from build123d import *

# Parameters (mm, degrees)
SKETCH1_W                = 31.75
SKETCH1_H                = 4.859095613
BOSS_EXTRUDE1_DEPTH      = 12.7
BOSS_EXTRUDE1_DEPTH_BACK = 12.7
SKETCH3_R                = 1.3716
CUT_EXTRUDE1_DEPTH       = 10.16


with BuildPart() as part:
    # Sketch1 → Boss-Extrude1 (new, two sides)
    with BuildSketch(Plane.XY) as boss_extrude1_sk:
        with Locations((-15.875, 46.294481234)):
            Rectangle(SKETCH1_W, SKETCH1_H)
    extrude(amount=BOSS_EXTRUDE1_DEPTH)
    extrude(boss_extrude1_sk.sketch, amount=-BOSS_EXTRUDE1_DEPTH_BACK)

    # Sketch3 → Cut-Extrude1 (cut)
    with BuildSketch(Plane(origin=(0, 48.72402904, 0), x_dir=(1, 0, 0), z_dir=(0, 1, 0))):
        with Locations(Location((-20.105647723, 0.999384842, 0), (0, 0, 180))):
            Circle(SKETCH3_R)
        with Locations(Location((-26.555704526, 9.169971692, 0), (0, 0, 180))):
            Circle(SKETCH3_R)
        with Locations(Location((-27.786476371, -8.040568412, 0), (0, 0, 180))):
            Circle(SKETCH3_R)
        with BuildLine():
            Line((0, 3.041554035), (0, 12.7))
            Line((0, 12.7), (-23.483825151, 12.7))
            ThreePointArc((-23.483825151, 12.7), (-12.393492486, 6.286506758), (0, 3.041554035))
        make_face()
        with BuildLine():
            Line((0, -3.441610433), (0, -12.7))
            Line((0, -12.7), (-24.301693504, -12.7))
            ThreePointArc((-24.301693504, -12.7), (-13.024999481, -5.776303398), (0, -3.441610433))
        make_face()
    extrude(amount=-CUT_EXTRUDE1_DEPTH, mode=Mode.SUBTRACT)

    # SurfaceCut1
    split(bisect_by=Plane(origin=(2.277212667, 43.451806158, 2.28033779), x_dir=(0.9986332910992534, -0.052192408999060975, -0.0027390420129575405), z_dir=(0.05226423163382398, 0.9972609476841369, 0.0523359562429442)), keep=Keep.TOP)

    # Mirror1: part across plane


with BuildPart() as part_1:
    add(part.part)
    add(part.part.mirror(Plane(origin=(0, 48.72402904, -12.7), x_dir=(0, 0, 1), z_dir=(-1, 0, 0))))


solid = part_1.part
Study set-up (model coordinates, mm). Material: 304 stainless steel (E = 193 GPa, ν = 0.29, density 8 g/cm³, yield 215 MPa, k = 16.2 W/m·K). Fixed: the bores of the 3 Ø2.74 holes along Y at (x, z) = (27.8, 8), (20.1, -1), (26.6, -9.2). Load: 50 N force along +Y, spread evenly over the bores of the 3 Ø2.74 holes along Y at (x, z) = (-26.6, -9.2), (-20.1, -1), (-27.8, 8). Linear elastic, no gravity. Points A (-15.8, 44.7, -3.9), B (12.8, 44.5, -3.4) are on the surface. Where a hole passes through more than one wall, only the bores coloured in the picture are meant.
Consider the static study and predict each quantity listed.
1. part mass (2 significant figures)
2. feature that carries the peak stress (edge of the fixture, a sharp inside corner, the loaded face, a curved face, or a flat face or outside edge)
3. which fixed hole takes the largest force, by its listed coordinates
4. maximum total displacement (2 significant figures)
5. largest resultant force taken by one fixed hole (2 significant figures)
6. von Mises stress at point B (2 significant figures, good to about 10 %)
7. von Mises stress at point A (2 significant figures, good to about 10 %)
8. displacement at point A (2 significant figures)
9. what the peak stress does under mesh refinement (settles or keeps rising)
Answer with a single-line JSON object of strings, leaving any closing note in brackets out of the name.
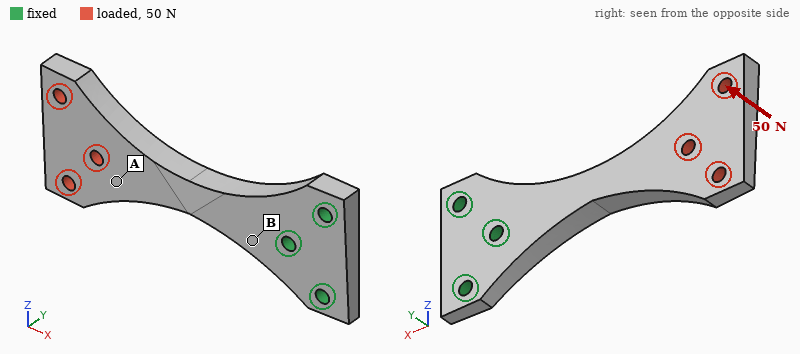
{"part mass": "31 g", "feature that carries the peak stress": "edge of the fixture", "which fixed hole takes the largest force, by its listed coordinates": "(20.1, -1)", "maximum total displacement": "0.13 mm", "largest resultant force taken by one fixed hole": "160 N", "von Mises stress at point B": "48 MPa", "von Mises stress at point A": "10 MPa", "displacement at point A": "0.073 mm", "what the peak stress does under mesh refinement": "keeps rising"}
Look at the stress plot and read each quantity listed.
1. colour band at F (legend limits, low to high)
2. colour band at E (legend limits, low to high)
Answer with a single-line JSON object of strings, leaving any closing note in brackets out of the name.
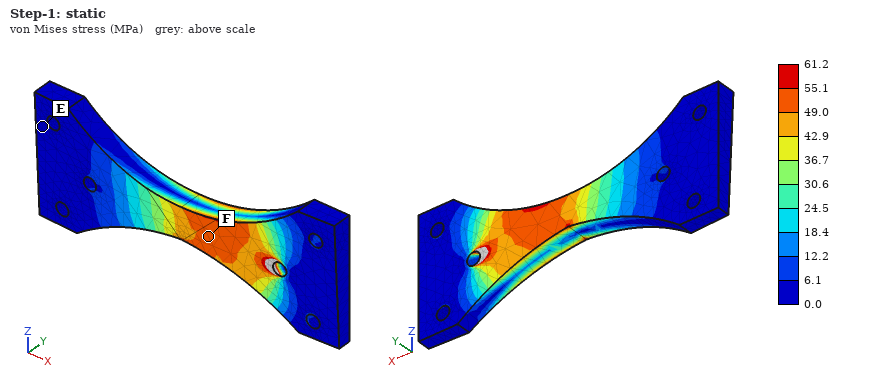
{"colour band at F": "49.0 to 55.1 MPa", "colour band at E": "0.0 to 6.1 MPa"}
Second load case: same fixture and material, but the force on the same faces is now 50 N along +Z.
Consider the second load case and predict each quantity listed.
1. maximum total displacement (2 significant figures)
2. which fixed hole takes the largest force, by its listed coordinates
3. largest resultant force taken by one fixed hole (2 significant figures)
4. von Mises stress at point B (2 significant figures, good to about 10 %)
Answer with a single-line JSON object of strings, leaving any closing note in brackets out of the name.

{"maximum total displacement": "36 µm", "which fixed hole takes the largest force, by its listed coordinates": "(27.8, 8)", "largest resultant force taken by one fixed hole": "130 N", "von Mises stress at point B": "12 MPa"}
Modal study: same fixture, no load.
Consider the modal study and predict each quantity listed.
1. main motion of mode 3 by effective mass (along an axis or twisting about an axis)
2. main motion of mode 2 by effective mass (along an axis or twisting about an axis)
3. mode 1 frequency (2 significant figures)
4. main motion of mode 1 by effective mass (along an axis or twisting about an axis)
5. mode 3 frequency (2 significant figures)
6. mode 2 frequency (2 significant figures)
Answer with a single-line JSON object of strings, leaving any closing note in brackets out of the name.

{"main motion of mode 3 by effective mass": "twisting about X", "main motion of mode 2 by effective mass": "along Z", "mode 1 frequency": "1000 Hz", "main motion of mode 1 by effective mass": "along Y", "mode 3 frequency": "4300 Hz", "mode 2 frequency": "2000 Hz"}
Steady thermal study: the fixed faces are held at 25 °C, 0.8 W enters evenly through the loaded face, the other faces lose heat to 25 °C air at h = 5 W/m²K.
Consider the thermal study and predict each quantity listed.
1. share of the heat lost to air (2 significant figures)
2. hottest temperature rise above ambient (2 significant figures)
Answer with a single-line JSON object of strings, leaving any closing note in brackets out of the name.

{"share of the heat lost to air": "29 %", "hottest temperature rise above ambient": "37 K"}
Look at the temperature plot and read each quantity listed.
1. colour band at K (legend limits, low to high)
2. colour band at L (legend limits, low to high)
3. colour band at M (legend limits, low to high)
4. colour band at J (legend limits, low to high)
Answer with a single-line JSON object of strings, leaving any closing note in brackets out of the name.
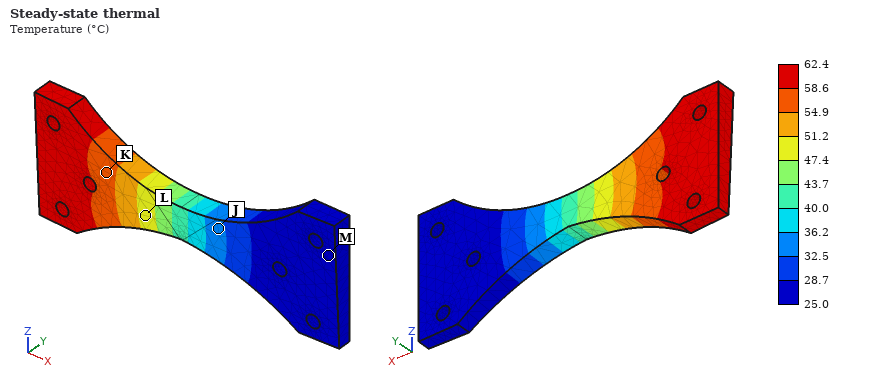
{"colour band at K": "54.9 to 58.6 °C", "colour band at L": "47.4 to 51.2 °C", "colour band at M": "25.0 to 28.7 °C", "colour band at J": "32.5 to 36.2 °C"}
